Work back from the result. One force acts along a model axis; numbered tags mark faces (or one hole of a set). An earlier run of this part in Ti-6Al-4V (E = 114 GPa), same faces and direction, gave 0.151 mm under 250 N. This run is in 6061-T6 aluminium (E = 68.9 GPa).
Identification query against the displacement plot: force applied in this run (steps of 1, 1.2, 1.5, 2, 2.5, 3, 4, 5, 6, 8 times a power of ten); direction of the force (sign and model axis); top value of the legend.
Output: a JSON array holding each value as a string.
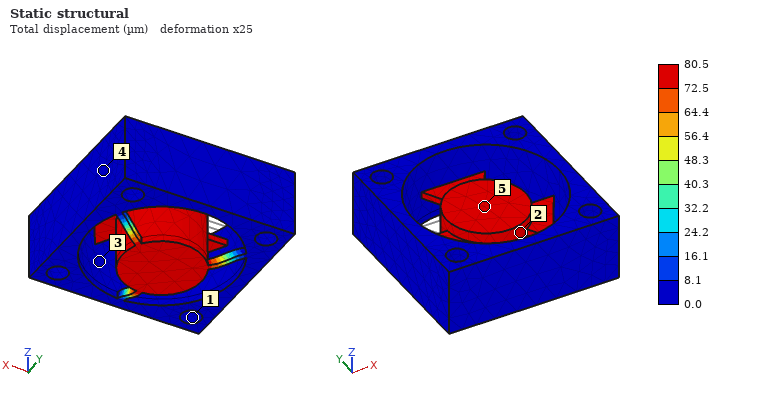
["80 N", "-Z", "80.5 µm"]
